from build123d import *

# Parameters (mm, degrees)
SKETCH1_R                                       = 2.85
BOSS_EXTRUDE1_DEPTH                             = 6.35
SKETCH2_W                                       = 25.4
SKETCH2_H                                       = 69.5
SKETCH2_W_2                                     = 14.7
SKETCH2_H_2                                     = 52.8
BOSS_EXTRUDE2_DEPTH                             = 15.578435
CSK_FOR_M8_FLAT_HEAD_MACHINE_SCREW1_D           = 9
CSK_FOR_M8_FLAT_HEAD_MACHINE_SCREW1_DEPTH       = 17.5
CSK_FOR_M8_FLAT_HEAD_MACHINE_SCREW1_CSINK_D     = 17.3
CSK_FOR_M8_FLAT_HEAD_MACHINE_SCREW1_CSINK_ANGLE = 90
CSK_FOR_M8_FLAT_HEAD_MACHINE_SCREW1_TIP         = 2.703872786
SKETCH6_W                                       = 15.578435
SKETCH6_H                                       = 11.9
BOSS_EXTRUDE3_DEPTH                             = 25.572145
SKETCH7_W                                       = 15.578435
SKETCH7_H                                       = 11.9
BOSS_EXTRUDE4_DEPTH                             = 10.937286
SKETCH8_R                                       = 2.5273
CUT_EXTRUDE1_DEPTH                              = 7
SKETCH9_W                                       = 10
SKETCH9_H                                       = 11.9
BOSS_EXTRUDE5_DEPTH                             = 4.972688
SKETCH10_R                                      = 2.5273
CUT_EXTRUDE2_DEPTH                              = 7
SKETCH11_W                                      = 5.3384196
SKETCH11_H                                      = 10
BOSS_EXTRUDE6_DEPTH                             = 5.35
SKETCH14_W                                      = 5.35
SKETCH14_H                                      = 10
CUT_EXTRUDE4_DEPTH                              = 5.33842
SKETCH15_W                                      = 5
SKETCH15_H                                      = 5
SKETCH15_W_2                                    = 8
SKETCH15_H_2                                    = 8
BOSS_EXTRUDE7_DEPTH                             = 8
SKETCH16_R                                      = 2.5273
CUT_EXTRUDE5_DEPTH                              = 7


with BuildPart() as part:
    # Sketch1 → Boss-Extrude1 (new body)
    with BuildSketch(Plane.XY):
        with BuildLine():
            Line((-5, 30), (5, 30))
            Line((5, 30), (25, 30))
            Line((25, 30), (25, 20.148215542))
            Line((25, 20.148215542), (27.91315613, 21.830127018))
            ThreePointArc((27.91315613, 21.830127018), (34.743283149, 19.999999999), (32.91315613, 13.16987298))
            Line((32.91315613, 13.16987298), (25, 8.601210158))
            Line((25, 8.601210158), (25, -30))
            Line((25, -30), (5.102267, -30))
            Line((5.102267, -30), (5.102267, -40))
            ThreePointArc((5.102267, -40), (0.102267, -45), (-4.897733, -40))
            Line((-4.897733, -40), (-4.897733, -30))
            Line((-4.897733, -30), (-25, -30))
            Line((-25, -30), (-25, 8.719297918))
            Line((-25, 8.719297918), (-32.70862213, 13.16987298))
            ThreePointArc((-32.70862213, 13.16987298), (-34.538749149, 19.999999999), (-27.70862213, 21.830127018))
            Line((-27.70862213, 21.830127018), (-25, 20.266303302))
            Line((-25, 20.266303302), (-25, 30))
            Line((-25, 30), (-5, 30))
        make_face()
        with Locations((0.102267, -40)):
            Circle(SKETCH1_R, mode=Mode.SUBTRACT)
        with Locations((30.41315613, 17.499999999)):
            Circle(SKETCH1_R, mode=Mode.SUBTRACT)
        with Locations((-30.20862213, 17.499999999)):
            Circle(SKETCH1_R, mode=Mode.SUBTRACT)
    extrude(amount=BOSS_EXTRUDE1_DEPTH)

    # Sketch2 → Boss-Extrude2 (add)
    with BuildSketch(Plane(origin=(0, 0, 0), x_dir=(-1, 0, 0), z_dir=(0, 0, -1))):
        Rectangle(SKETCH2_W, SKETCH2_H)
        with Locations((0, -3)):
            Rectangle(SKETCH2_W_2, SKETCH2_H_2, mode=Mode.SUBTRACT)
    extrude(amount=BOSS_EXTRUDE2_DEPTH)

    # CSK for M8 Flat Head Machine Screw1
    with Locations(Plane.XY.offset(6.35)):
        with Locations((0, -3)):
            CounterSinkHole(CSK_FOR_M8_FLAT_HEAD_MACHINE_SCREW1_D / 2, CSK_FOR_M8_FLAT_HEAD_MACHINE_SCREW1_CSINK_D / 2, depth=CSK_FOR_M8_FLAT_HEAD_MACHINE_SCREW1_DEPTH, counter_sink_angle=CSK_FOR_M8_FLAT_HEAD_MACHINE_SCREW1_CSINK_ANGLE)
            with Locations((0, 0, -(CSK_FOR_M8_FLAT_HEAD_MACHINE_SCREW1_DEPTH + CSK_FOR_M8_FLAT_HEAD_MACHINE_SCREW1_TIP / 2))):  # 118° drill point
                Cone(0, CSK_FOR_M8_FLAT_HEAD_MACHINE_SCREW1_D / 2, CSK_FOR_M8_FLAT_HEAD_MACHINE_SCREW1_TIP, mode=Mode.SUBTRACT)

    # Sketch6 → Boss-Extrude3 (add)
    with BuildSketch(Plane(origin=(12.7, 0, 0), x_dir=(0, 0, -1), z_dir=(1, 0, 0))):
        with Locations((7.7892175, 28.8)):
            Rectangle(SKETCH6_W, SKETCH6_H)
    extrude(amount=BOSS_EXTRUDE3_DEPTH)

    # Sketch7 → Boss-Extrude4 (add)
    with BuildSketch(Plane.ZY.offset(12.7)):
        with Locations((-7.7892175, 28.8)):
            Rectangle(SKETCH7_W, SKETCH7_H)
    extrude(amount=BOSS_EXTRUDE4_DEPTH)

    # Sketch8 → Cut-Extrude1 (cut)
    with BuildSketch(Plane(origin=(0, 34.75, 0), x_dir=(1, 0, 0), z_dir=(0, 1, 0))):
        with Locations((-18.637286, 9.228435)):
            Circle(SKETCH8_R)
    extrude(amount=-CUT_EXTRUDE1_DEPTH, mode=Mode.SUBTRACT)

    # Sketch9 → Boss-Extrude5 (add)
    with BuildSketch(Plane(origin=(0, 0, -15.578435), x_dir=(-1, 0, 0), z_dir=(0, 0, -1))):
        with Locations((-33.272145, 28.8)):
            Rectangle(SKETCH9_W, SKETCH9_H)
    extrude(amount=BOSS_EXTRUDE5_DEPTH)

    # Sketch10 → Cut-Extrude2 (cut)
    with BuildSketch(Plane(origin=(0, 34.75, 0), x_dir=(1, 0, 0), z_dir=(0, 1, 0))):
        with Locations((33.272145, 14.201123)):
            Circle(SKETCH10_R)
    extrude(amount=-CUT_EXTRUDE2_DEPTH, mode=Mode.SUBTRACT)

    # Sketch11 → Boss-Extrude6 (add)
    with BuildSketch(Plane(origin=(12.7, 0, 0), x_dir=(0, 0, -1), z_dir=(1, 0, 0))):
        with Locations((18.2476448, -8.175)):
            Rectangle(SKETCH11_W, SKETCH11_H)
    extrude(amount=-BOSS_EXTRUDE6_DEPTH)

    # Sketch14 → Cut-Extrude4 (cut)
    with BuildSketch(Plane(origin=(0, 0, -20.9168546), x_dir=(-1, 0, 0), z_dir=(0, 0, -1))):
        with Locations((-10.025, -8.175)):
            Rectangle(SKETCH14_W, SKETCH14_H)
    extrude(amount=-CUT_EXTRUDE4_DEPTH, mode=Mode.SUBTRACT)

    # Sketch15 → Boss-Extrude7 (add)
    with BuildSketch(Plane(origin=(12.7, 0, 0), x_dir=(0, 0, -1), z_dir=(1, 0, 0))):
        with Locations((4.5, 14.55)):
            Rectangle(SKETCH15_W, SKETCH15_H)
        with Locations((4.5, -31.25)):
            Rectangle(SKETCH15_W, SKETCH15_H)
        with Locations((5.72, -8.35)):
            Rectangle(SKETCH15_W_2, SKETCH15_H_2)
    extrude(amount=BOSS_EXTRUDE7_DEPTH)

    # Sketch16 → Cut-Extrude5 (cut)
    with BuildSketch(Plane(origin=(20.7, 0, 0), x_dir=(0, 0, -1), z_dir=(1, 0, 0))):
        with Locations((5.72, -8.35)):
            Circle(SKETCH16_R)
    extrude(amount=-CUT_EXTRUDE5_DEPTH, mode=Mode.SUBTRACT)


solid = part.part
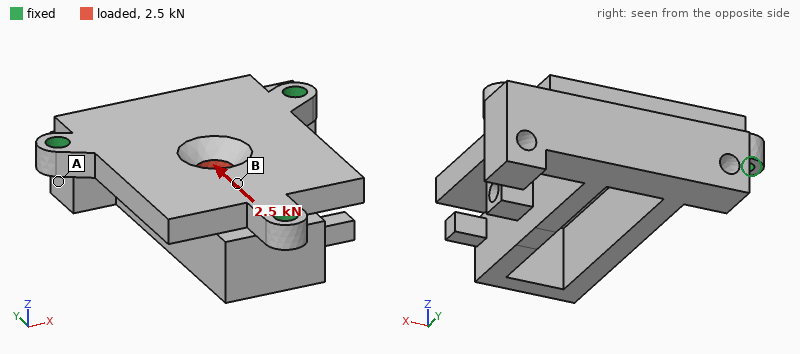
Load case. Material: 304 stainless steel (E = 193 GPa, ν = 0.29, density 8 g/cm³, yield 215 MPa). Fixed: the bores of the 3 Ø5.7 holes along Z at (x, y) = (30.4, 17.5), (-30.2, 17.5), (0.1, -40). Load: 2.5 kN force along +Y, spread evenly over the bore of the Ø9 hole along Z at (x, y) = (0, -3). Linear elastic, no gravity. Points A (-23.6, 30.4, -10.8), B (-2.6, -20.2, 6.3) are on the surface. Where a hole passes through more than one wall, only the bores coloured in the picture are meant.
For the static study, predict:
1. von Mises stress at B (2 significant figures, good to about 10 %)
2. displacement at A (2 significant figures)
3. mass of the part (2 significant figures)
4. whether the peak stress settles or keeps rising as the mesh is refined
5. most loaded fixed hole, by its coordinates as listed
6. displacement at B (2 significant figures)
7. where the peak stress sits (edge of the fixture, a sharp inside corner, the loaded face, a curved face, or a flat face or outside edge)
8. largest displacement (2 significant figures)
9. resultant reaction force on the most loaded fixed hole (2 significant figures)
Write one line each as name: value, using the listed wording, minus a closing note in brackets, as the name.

von Mises stress at B: 10 MPa
displacement at A: 1.5 µm
mass of the part: 350 g
whether the peak stress settles or keeps rising as the mesh is refined: keeps rising
most loaded fixed hole, by its coordinates as listed: (0.1, -40)
displacement at B: 1.2 µm
where the peak stress sits: a sharp inside corner
largest displacement: 3.3 µm
resultant reaction force on the most loaded fixed hole: 1.2 kN
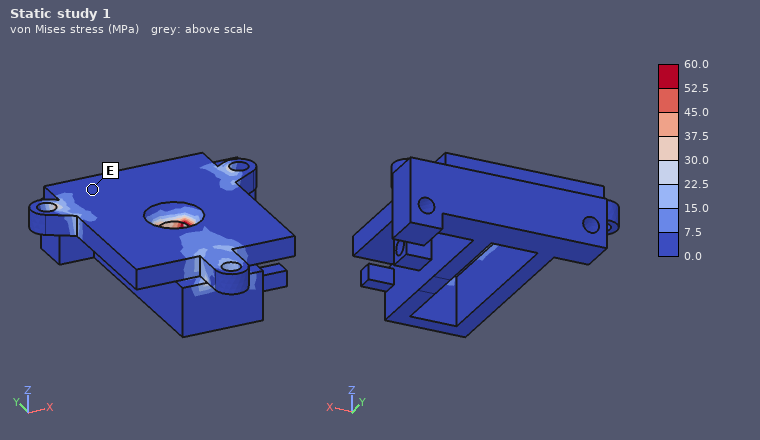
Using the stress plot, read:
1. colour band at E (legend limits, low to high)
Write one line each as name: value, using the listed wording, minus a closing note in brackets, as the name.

colour band at E: 0.0 to 7.5 MPa
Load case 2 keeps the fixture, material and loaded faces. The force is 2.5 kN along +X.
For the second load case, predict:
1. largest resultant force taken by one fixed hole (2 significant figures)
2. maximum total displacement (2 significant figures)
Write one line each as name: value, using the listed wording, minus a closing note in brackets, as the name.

largest resultant force taken by one fixed hole: 1.1 kN
maximum total displacement: 3.6 µm
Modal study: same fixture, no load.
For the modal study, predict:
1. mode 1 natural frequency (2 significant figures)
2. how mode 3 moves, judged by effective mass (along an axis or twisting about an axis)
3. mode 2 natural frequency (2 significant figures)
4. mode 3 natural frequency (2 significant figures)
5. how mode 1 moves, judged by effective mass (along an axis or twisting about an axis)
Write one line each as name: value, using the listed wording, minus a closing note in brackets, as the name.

mode 1 natural frequency: 5100 Hz
how mode 3 moves, judged by effective mass: along Z
mode 2 natural frequency: 5500 Hz
mode 3 natural frequency: 7100 Hz
how mode 1 moves, judged by effective mass: along Z
